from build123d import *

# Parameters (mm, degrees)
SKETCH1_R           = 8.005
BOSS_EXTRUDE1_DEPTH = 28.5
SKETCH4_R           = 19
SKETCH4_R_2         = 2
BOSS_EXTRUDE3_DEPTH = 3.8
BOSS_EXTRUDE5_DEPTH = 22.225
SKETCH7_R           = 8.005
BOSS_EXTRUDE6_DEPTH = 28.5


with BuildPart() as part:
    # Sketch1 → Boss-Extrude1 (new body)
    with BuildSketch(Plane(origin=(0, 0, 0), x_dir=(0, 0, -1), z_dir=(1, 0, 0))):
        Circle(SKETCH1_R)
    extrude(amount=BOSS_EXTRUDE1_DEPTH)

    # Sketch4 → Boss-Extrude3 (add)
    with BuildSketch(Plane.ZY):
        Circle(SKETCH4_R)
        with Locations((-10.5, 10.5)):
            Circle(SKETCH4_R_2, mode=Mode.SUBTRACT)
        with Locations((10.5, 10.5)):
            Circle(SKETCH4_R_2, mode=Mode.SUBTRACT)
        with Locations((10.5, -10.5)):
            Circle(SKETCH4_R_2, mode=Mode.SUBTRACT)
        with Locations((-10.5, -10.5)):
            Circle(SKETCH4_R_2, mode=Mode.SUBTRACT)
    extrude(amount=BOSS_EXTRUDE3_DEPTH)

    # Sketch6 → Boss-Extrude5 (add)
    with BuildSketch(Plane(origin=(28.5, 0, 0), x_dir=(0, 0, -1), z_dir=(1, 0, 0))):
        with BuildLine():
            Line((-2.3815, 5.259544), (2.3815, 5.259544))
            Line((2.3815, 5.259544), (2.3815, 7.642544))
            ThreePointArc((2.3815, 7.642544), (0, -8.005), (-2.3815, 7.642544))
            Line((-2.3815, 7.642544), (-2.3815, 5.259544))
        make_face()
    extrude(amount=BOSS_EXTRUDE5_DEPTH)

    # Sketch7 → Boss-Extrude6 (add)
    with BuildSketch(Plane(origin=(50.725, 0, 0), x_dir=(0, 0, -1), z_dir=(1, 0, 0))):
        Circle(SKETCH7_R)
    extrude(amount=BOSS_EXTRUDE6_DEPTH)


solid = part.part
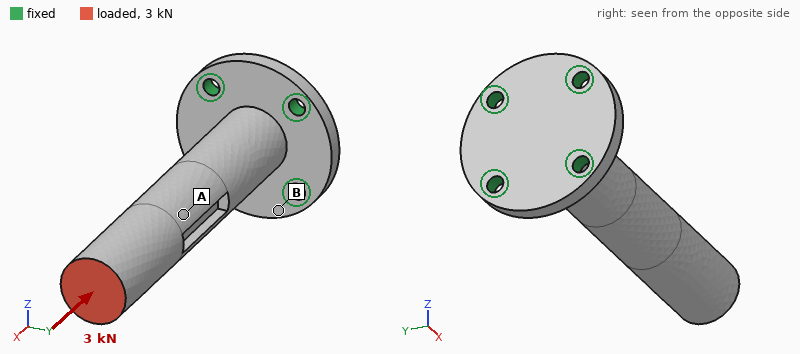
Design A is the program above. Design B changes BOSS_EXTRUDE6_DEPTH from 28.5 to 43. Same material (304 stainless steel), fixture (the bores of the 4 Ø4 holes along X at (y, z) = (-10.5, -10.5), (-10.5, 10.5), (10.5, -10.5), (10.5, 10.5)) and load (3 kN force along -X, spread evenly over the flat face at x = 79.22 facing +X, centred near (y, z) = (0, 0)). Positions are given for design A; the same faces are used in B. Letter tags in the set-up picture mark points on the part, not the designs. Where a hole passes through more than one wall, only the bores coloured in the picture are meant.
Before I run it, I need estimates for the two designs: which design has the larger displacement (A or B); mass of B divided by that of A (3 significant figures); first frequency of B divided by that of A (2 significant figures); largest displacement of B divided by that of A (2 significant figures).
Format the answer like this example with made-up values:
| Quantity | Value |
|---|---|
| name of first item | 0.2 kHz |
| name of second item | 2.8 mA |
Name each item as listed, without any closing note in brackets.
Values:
| Quantity | Value |
|---|---|
| which design has the larger displacement | B |
| mass of B divided by that of A | 1.15 |
| first frequency of B divided by that of A | 0.73 |
| largest displacement of B divided by that of A | 1.1 |
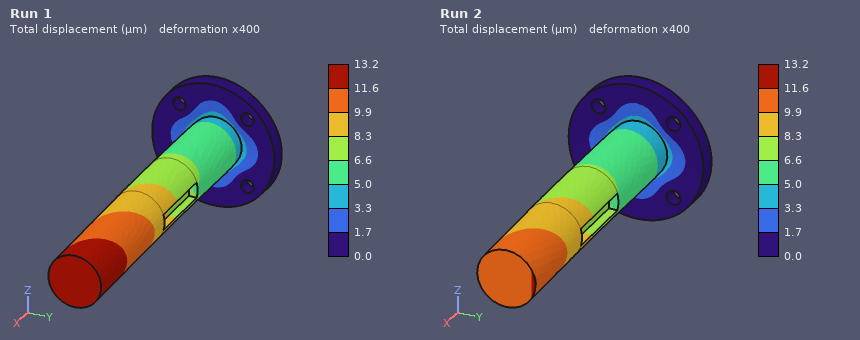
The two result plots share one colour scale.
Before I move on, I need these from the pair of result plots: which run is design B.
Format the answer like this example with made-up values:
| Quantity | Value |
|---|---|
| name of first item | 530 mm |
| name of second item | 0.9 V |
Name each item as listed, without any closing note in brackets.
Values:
| Quantity | Value |
|---|---|
| which run is design B | Run 1 |
